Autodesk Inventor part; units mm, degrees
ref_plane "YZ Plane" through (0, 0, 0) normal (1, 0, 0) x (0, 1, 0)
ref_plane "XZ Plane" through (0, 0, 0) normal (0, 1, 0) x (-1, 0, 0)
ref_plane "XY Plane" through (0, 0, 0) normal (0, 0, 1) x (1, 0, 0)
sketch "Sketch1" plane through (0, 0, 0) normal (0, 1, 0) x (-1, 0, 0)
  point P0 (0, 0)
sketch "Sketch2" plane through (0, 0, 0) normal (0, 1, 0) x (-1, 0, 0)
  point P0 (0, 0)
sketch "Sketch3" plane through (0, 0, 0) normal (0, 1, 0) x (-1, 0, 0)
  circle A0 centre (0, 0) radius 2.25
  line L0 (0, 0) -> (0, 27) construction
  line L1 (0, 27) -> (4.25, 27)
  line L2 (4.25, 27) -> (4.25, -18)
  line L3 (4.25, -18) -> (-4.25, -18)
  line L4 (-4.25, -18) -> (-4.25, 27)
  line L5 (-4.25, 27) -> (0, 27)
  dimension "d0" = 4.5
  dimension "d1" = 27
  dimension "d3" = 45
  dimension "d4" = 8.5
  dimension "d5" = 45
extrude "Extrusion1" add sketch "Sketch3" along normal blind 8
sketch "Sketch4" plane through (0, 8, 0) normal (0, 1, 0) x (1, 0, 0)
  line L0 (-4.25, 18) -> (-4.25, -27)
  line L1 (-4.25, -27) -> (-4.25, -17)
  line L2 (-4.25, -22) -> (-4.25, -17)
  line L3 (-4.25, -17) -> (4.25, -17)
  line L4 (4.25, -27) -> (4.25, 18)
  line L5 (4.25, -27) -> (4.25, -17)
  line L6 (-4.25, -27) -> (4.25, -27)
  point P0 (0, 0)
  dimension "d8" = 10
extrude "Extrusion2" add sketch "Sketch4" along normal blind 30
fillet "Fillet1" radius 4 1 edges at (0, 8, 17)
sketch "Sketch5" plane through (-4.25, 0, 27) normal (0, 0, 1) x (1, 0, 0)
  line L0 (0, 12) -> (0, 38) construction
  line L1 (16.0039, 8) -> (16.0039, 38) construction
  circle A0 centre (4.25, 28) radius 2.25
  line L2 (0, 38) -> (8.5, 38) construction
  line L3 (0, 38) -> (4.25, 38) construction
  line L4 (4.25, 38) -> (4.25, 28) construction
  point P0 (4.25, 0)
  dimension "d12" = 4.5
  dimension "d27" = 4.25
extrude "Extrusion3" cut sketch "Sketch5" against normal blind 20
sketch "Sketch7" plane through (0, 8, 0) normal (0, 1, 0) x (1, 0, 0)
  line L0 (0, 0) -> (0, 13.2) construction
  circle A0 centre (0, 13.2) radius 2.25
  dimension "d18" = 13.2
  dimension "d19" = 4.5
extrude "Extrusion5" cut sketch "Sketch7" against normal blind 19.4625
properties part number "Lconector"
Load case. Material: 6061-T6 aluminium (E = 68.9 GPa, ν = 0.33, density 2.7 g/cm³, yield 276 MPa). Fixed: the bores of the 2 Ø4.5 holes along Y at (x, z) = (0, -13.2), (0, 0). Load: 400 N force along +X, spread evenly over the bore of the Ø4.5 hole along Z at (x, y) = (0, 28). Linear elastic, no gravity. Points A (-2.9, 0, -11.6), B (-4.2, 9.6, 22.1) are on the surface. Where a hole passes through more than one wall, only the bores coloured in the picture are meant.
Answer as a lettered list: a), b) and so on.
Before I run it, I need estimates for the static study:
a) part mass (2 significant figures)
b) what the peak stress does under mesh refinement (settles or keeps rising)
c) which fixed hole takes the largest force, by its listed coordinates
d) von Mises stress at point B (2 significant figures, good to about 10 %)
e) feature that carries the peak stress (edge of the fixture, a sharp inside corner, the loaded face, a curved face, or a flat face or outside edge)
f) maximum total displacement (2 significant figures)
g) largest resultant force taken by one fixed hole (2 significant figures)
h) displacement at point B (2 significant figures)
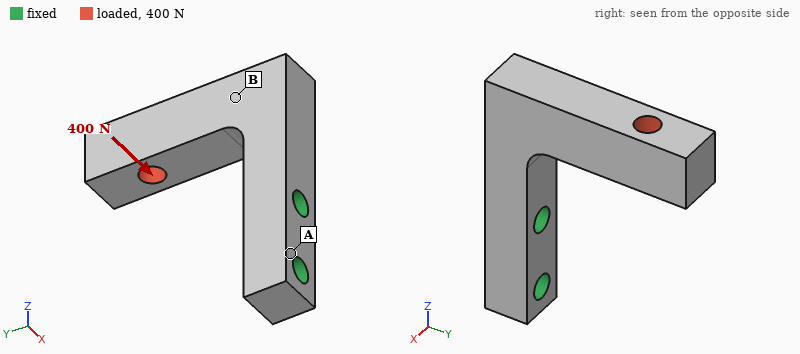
a) 14 g
b) keeps rising
c) (0, 0)
d) 50 MPa
e) edge of the fixture
f) 0.46 mm
g) 500 N
h) 0.12 mm
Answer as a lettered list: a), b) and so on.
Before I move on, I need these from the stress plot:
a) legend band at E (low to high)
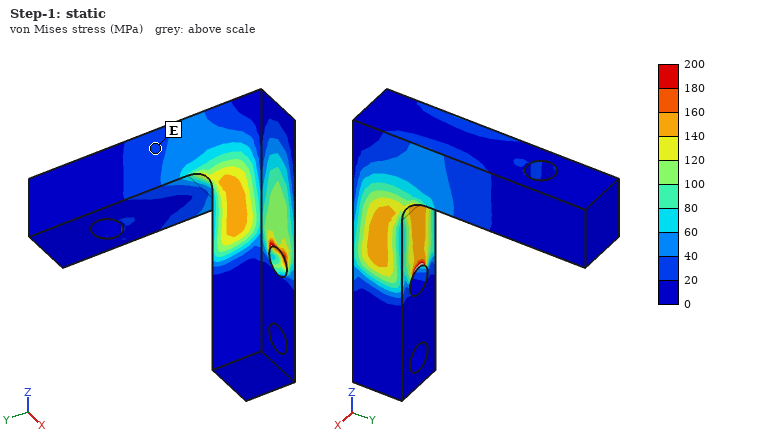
a) 20 to 40 MPa
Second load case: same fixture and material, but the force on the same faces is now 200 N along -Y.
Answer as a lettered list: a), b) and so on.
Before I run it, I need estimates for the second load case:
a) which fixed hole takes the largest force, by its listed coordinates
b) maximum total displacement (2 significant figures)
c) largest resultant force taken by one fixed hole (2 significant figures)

a) (0, 0)
b) 68 µm
c) 210 N
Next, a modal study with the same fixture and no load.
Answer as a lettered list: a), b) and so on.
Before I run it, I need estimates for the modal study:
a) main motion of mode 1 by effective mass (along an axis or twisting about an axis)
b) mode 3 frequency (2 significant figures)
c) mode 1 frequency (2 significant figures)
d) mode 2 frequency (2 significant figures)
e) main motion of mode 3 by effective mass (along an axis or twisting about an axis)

a) along X
b) 7200 Hz
c) 2500 Hz
d) 2800 Hz
e) along X
